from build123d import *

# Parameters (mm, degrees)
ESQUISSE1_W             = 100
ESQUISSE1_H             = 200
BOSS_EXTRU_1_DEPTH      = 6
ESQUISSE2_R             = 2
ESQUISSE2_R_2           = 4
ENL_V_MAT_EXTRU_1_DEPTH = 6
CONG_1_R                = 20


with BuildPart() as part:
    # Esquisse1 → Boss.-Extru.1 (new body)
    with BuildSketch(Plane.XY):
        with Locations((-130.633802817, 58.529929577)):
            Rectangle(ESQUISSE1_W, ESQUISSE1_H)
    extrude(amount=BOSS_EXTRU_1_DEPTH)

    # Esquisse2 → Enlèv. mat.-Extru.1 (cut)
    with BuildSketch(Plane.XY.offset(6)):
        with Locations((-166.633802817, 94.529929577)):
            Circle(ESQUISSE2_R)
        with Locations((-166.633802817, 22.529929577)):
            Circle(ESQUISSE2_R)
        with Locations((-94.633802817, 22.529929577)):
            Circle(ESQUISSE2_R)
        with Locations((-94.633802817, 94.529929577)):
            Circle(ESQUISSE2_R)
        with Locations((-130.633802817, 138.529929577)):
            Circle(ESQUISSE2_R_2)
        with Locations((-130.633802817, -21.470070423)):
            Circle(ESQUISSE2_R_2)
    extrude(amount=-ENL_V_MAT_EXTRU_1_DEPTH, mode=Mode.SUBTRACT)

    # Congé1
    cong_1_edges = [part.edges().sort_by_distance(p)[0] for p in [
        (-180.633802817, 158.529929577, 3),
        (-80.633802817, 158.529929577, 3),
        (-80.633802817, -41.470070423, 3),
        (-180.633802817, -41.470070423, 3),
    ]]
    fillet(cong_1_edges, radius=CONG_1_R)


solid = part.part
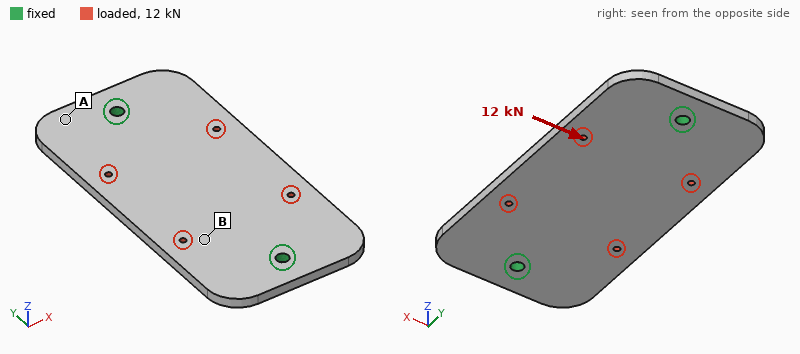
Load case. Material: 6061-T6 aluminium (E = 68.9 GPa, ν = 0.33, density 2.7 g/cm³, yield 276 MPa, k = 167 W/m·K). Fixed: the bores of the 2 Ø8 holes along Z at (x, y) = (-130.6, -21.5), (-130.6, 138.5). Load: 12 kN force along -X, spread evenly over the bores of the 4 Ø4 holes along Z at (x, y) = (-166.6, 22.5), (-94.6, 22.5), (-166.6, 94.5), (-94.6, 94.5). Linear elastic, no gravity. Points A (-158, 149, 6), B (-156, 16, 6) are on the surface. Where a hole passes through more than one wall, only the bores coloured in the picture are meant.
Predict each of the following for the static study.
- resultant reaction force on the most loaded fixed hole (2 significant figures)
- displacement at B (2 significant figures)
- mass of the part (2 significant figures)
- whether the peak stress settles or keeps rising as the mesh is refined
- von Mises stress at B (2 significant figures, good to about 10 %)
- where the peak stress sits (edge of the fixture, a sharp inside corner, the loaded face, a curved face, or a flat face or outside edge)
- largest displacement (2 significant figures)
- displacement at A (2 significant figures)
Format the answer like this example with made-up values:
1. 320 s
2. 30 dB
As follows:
1. 6.0 kN
2. 35 µm
3. 320 g
4. keeps rising
5. 23 MPa
6. edge of the fixture
7. 44 µm
8. 9.3 µm
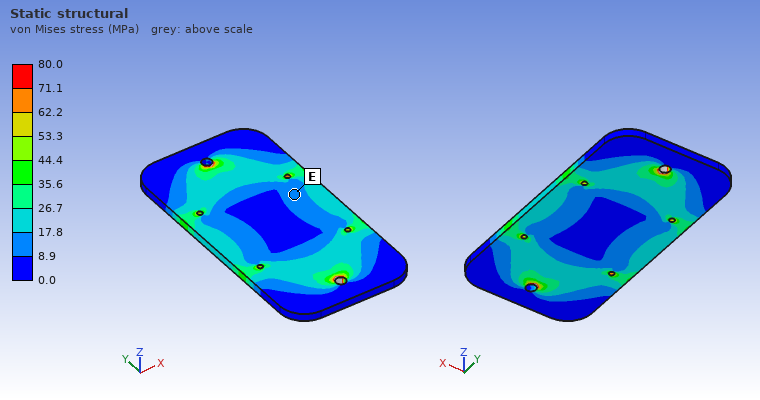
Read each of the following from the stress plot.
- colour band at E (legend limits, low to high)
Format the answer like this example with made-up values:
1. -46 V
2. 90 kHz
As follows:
1. 8.9 to 17.8 MPa
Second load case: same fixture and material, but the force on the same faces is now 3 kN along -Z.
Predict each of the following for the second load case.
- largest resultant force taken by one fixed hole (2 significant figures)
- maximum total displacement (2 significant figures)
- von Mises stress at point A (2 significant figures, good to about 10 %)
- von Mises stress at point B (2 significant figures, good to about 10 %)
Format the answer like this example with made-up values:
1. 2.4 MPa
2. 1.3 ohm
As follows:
1. 1.5 kN
2. 0.57 mm
3. 30 MPa
4. 28 MPa
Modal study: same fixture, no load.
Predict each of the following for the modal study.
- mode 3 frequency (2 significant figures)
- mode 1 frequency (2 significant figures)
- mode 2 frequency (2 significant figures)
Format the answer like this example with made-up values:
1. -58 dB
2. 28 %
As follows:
1. 2000 Hz
2. 980 Hz
3. 990 Hz
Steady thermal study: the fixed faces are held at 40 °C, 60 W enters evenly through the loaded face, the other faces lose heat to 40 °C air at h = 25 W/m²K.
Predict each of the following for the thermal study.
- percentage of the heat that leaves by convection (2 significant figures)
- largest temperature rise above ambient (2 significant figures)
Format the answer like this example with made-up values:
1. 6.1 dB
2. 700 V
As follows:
1. 21 %
2. 21 K
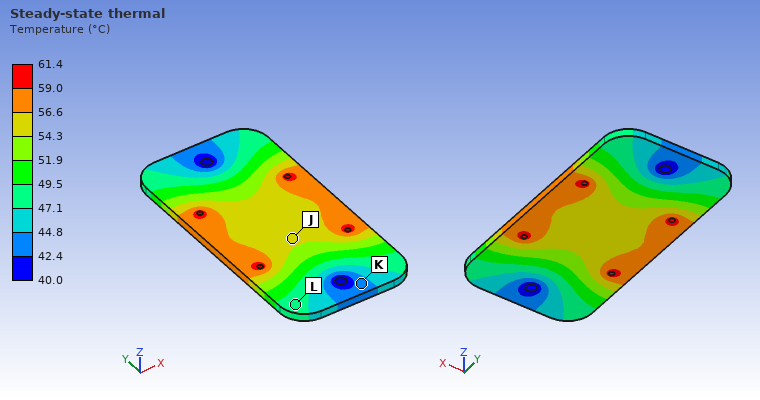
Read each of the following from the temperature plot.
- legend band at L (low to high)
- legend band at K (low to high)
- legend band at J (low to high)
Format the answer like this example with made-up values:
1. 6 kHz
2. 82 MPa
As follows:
1. 47.1 to 49.5 °C
2. 42.4 to 44.8 °C
3. 54.3 to 56.6 °C
